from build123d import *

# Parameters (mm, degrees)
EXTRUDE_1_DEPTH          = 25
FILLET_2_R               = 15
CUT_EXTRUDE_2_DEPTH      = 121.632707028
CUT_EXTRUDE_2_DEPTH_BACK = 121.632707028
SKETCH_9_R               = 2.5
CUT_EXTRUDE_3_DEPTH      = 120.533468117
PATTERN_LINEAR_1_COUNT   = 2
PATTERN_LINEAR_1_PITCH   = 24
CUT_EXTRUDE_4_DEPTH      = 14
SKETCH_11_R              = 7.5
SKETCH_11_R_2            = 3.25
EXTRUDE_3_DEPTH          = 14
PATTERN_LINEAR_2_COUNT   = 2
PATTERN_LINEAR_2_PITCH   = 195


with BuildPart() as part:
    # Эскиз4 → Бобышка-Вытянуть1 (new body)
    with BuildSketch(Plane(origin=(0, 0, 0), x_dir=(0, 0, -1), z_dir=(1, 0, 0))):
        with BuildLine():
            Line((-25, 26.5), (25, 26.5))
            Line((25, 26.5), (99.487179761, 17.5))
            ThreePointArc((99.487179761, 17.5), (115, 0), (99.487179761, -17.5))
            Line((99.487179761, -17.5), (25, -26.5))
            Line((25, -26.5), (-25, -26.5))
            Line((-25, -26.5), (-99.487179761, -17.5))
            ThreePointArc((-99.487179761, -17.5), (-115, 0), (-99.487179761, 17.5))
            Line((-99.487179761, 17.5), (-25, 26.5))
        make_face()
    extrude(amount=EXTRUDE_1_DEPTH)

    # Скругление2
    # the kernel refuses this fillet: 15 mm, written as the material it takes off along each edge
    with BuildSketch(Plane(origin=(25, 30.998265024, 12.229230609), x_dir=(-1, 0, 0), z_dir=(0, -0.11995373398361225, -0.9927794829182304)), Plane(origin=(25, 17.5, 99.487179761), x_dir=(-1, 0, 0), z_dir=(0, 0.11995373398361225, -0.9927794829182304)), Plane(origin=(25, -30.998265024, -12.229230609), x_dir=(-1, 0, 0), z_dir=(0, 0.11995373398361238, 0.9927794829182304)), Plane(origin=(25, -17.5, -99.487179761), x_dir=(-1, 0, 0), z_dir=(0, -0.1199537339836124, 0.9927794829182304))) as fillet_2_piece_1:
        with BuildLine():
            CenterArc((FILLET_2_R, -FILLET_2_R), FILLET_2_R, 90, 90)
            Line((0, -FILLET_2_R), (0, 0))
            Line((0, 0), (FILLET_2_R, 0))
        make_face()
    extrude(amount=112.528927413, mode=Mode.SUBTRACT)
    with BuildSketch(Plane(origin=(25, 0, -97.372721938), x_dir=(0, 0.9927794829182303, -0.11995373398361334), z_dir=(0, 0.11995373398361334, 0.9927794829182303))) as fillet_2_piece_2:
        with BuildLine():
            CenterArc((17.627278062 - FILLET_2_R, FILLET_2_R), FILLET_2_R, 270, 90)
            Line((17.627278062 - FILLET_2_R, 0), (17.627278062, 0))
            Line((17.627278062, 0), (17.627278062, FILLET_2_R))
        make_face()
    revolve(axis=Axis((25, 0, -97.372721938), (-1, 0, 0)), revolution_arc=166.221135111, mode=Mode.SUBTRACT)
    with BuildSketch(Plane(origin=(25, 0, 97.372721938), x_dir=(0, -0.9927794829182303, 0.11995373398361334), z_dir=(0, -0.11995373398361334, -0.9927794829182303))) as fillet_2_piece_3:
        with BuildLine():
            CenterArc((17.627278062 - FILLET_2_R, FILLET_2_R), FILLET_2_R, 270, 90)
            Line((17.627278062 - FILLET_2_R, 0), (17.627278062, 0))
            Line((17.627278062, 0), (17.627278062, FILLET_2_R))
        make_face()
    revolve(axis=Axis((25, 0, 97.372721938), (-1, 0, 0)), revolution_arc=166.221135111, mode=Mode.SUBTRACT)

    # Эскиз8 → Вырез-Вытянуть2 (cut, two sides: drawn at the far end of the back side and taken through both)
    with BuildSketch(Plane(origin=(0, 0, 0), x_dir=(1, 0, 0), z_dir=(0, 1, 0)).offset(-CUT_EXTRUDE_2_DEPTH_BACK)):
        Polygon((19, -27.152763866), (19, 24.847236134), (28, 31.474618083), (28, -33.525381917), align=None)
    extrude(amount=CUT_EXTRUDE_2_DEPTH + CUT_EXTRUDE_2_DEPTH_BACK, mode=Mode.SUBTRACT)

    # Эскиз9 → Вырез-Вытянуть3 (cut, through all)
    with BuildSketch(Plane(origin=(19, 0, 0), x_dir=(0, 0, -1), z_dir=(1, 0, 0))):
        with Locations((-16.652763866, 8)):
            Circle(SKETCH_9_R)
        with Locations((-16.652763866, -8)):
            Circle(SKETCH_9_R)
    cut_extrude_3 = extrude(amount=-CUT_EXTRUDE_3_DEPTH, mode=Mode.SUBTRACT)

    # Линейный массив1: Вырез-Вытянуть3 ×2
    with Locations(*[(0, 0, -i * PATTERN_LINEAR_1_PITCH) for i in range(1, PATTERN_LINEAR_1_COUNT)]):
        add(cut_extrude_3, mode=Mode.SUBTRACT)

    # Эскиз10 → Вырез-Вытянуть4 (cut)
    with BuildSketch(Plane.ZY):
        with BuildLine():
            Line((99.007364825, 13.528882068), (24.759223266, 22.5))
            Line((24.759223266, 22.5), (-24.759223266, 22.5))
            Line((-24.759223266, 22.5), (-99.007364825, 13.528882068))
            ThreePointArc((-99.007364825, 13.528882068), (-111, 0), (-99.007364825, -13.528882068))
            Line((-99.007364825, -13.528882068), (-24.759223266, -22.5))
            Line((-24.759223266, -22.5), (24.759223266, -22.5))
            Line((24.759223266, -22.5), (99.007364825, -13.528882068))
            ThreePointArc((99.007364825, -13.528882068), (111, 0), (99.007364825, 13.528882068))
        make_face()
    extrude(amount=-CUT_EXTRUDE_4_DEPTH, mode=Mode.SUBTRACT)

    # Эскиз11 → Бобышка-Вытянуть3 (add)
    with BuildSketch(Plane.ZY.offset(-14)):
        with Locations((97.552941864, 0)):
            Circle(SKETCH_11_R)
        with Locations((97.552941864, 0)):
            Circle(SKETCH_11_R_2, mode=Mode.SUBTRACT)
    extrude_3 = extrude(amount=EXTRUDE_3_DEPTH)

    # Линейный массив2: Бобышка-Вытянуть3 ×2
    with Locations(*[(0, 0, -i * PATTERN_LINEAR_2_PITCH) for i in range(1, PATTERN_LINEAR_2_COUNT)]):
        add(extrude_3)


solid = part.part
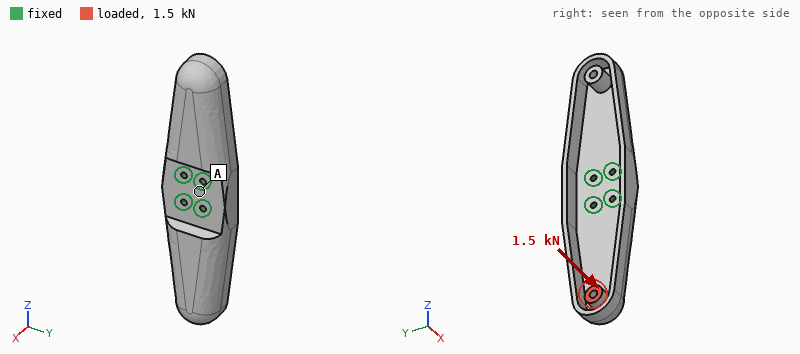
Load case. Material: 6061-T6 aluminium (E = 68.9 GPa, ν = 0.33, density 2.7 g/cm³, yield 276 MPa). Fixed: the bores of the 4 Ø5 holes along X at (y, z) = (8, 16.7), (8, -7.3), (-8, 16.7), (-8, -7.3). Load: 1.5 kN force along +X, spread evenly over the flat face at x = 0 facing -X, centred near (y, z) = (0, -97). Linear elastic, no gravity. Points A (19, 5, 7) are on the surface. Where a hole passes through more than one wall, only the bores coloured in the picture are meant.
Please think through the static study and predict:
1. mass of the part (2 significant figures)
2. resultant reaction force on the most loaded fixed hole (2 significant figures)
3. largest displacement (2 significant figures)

280 g
2.8 kN
1.3 mm
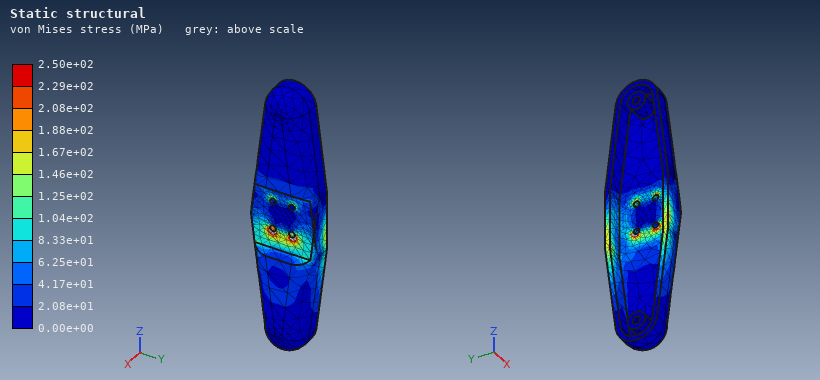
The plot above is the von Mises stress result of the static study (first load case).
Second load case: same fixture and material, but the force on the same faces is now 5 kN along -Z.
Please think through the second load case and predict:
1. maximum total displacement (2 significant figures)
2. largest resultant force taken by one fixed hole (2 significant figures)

0.89 mm
1.9 kN
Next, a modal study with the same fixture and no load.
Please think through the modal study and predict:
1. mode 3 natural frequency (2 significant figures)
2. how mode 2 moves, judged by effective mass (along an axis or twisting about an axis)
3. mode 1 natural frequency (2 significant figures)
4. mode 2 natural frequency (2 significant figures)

2100 Hz
along X
720 Hz
1100 Hz
